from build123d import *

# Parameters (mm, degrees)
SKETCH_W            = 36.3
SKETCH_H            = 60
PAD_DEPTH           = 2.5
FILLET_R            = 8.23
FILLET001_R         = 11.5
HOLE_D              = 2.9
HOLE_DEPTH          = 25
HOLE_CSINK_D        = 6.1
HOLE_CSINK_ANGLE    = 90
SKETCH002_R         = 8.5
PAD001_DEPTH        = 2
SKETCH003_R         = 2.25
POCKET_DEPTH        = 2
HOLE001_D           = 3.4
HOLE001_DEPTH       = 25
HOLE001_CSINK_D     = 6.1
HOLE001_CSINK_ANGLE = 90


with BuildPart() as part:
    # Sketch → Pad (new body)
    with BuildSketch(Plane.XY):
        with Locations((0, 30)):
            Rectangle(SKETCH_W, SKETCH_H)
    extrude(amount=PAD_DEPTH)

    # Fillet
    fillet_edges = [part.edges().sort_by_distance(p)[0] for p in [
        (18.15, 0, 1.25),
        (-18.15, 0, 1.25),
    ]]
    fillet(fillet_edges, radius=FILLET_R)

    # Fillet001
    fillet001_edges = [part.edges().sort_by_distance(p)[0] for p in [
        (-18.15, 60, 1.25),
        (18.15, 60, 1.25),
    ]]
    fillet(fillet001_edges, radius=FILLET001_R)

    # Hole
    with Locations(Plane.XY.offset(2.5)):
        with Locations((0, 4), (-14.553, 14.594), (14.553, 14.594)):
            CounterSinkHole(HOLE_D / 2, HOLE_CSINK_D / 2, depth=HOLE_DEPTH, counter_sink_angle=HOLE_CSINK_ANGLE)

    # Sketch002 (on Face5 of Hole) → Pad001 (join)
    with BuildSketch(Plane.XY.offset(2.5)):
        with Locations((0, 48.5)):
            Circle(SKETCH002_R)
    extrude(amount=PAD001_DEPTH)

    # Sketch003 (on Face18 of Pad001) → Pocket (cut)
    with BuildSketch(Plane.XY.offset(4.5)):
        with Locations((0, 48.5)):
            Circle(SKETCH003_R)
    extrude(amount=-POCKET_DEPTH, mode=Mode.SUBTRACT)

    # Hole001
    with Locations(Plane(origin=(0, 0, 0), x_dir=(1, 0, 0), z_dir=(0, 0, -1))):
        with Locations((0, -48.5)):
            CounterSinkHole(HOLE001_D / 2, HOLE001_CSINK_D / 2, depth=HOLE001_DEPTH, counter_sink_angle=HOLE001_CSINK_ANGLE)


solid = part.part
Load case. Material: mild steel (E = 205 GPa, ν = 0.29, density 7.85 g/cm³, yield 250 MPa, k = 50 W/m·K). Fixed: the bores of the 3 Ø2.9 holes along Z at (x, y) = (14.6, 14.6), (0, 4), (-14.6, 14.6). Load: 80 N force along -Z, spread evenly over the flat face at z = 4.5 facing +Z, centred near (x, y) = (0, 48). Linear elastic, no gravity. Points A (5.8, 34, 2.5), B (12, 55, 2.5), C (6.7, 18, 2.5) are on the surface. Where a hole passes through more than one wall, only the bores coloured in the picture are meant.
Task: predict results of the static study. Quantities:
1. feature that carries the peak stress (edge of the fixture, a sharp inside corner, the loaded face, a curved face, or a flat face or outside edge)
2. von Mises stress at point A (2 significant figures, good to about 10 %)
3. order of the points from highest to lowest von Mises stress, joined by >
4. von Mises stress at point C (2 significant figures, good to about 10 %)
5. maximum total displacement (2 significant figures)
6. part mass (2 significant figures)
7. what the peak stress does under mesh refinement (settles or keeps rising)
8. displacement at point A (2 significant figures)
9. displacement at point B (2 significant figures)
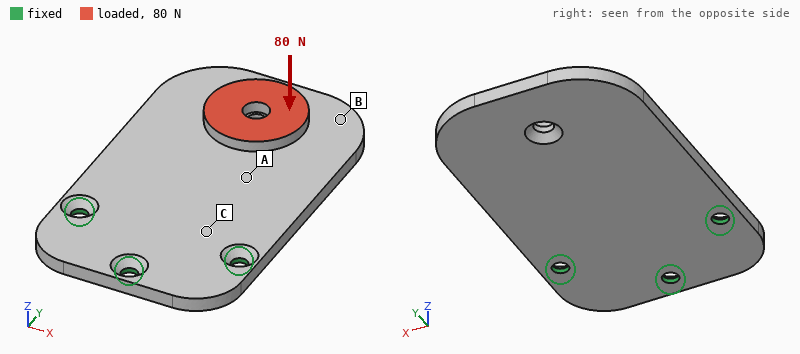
edge of the fixture
32 MPa
C > A > B
66 MPa
0.22 mm
43 g
keeps rising
0.069 mm
0.19 mm
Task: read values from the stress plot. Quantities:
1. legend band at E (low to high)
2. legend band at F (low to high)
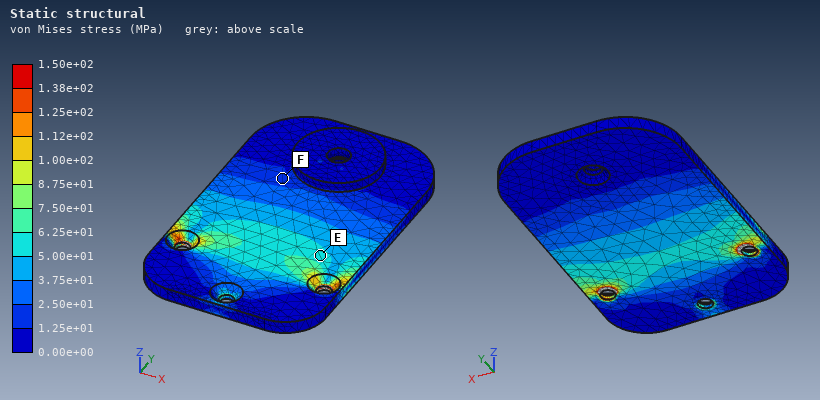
5.00e+01 to 6.25e+01 MPa
1.25e+01 to 2.50e+01 MPa
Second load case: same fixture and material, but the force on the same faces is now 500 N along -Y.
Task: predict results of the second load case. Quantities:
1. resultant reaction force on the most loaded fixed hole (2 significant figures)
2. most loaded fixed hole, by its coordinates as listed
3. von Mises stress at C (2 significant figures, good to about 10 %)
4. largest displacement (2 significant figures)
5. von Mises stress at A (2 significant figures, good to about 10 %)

270 N
(0, 4)
49 MPa
0.19 mm
48 MPa
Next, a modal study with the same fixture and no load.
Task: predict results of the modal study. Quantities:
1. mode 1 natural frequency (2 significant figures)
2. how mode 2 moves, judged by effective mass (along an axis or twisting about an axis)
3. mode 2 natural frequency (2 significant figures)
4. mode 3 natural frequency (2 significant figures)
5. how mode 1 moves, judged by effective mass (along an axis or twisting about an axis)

830 Hz
twisting about Y
3200 Hz
5600 Hz
along Z
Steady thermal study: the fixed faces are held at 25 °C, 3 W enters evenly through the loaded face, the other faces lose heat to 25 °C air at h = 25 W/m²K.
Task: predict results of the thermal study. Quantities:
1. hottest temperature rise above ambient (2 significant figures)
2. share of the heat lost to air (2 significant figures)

20 K
34 %
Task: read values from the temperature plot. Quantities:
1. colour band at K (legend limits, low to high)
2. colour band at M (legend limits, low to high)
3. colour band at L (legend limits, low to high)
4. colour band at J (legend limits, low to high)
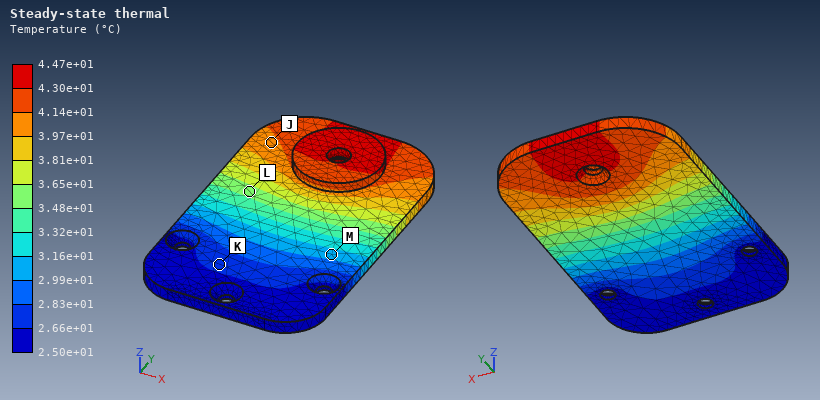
2.66e+01 to 2.83e+01 °C
2.99e+01 to 3.16e+01 °C
3.48e+01 to 3.65e+01 °C
3.97e+01 to 4.14e+01 °C
